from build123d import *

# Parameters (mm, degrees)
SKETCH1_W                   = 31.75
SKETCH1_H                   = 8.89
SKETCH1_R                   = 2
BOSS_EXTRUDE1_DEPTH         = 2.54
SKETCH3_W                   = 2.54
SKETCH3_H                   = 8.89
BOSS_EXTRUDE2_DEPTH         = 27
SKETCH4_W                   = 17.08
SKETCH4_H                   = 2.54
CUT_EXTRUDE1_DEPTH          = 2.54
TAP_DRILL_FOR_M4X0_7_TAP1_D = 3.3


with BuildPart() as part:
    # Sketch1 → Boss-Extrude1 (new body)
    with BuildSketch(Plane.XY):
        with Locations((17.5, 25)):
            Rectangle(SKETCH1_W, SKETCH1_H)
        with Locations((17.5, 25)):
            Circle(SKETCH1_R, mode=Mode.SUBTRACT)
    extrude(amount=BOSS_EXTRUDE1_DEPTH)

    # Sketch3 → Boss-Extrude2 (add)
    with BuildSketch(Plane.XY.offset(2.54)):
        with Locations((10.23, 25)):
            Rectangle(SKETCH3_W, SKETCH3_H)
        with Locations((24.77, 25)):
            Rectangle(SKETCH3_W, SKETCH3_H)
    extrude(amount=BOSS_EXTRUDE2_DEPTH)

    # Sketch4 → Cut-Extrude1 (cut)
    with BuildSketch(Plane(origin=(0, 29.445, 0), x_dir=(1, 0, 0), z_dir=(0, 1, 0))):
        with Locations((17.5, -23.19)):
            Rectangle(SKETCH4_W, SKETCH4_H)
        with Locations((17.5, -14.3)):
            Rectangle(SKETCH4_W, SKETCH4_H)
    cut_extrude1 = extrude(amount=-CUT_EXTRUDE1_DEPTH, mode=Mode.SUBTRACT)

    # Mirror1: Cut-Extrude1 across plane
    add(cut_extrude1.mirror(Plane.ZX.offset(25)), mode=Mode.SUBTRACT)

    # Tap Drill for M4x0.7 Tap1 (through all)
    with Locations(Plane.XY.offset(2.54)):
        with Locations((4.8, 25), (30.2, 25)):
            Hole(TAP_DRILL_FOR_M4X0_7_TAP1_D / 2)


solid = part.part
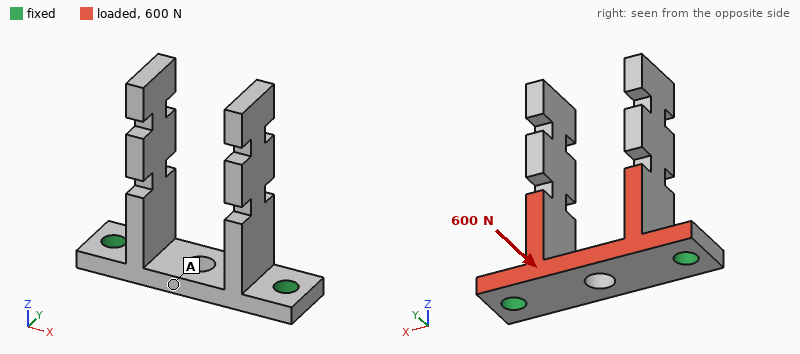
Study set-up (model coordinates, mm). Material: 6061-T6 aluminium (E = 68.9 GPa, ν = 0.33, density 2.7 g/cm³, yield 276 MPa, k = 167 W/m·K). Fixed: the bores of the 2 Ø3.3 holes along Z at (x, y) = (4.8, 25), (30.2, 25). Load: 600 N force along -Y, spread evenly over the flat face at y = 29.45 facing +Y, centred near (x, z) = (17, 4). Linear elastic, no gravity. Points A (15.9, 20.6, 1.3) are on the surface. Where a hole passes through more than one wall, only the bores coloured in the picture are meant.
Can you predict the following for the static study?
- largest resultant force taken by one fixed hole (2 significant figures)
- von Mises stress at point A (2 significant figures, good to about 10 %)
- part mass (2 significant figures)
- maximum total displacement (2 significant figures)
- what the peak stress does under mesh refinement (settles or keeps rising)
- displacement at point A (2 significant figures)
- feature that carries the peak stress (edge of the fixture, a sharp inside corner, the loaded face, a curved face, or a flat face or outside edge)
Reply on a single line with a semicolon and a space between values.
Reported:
300 N; 18 MPa; 4.7 g; 69 µm; keeps rising; 11 µm; edge of the fixture
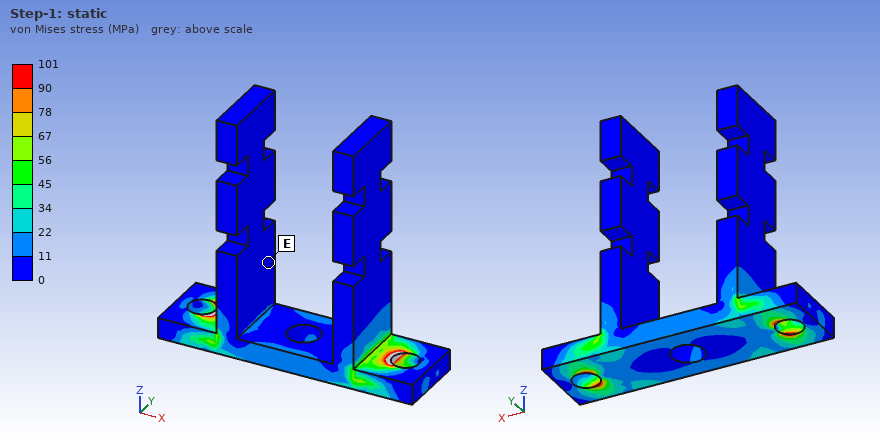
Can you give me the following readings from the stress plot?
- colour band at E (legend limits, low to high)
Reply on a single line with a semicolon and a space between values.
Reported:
0 to 11 MPa
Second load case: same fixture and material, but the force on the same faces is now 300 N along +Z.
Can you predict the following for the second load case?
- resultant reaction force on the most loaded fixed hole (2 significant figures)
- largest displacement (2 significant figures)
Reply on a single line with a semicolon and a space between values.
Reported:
150 N; 62 µm
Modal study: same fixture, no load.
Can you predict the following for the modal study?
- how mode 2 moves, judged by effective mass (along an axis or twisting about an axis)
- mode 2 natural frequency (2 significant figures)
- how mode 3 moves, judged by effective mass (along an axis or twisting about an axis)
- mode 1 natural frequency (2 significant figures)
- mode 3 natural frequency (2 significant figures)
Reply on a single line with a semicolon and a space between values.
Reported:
along X; 2500 Hz; along Y; 2300 Hz; 3800 Hz
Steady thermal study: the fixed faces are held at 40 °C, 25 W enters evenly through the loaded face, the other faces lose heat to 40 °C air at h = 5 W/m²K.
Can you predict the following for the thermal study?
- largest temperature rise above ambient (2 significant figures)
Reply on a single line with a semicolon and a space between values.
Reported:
22 K
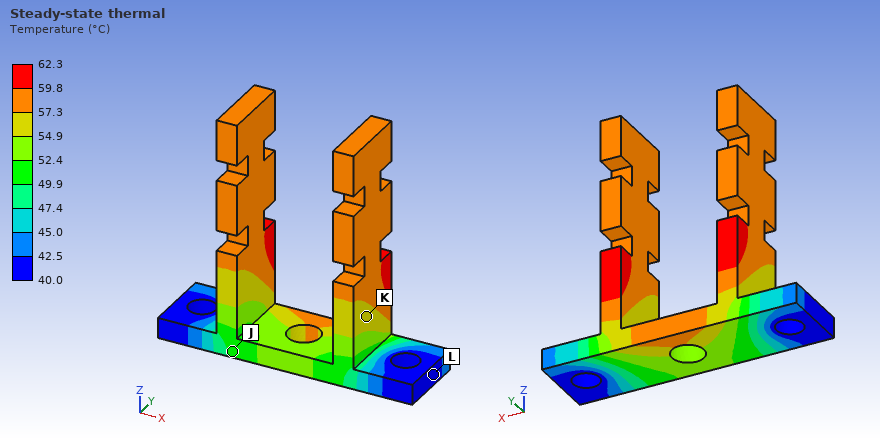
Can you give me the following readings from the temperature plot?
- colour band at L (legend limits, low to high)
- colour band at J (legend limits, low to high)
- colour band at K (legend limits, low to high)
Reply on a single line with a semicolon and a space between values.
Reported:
40.0 to 42.5 °C; 49.9 to 52.4 °C; 54.9 to 57.3 °C
